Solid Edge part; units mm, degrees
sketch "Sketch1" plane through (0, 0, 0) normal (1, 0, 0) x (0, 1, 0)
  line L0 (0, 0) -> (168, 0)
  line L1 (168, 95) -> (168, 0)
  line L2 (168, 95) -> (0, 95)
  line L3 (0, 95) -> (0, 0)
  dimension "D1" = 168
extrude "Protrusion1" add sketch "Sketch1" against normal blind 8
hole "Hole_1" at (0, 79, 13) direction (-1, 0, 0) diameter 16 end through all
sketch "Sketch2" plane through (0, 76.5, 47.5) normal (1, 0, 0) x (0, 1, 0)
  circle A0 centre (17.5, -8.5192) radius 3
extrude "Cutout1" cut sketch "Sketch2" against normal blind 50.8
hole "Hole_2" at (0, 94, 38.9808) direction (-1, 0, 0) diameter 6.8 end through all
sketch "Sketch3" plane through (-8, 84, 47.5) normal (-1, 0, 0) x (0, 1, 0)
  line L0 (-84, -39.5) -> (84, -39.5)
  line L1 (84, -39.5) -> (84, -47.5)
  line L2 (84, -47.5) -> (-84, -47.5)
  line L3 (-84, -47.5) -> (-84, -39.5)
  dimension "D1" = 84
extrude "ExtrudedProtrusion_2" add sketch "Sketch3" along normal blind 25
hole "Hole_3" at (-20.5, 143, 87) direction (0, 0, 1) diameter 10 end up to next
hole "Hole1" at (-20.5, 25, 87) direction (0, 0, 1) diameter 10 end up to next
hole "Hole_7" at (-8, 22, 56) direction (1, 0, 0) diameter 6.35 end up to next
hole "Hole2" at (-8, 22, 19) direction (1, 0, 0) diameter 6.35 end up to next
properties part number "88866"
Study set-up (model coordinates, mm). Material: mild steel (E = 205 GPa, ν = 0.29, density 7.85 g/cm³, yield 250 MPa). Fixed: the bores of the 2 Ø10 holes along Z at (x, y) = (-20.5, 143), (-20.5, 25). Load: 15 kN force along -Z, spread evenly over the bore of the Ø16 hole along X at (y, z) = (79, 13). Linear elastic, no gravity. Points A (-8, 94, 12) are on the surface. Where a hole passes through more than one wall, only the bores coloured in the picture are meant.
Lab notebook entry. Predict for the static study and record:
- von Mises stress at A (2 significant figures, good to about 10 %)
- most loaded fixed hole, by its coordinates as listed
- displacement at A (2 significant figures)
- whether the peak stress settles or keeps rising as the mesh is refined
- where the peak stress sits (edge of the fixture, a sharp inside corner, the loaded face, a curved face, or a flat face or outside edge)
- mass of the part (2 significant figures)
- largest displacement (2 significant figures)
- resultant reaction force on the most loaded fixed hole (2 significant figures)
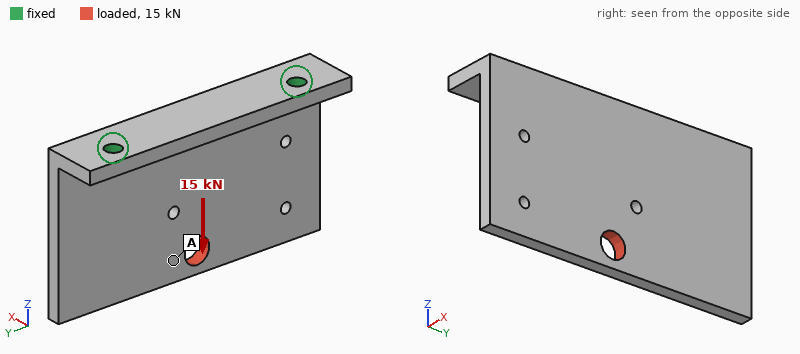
40 MPa
(-20.5, 25)
0.17 mm
keeps rising
edge of the fixture
1.2 kg
0.21 mm
8.3 kN
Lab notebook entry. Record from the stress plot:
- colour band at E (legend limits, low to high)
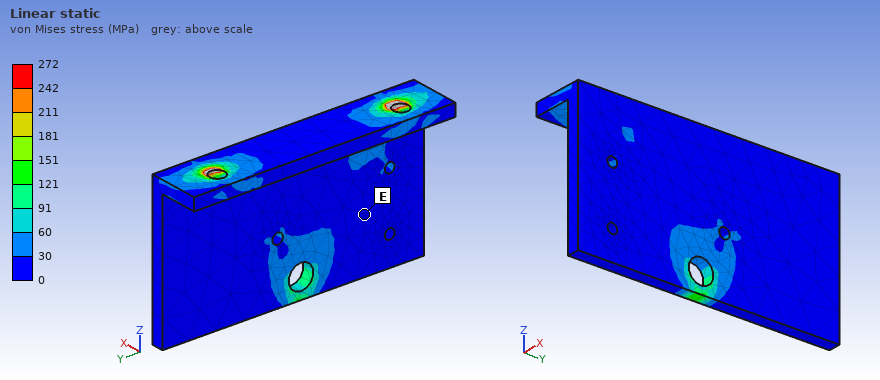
0 to 30 MPa
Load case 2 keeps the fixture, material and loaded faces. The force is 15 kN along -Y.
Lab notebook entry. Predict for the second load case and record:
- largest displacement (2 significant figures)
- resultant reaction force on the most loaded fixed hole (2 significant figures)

0.14 mm
12 kN
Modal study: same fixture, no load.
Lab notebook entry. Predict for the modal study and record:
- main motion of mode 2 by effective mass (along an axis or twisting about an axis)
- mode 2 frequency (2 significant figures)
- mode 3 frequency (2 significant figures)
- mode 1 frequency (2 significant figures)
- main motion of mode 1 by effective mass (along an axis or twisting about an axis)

twisting about Z
1100 Hz
2400 Hz
580 Hz
along X
